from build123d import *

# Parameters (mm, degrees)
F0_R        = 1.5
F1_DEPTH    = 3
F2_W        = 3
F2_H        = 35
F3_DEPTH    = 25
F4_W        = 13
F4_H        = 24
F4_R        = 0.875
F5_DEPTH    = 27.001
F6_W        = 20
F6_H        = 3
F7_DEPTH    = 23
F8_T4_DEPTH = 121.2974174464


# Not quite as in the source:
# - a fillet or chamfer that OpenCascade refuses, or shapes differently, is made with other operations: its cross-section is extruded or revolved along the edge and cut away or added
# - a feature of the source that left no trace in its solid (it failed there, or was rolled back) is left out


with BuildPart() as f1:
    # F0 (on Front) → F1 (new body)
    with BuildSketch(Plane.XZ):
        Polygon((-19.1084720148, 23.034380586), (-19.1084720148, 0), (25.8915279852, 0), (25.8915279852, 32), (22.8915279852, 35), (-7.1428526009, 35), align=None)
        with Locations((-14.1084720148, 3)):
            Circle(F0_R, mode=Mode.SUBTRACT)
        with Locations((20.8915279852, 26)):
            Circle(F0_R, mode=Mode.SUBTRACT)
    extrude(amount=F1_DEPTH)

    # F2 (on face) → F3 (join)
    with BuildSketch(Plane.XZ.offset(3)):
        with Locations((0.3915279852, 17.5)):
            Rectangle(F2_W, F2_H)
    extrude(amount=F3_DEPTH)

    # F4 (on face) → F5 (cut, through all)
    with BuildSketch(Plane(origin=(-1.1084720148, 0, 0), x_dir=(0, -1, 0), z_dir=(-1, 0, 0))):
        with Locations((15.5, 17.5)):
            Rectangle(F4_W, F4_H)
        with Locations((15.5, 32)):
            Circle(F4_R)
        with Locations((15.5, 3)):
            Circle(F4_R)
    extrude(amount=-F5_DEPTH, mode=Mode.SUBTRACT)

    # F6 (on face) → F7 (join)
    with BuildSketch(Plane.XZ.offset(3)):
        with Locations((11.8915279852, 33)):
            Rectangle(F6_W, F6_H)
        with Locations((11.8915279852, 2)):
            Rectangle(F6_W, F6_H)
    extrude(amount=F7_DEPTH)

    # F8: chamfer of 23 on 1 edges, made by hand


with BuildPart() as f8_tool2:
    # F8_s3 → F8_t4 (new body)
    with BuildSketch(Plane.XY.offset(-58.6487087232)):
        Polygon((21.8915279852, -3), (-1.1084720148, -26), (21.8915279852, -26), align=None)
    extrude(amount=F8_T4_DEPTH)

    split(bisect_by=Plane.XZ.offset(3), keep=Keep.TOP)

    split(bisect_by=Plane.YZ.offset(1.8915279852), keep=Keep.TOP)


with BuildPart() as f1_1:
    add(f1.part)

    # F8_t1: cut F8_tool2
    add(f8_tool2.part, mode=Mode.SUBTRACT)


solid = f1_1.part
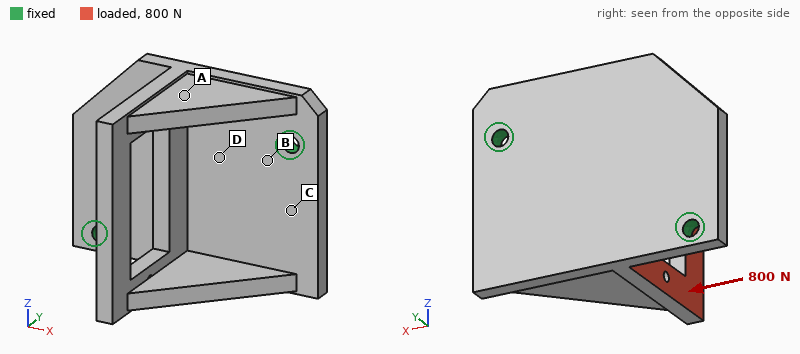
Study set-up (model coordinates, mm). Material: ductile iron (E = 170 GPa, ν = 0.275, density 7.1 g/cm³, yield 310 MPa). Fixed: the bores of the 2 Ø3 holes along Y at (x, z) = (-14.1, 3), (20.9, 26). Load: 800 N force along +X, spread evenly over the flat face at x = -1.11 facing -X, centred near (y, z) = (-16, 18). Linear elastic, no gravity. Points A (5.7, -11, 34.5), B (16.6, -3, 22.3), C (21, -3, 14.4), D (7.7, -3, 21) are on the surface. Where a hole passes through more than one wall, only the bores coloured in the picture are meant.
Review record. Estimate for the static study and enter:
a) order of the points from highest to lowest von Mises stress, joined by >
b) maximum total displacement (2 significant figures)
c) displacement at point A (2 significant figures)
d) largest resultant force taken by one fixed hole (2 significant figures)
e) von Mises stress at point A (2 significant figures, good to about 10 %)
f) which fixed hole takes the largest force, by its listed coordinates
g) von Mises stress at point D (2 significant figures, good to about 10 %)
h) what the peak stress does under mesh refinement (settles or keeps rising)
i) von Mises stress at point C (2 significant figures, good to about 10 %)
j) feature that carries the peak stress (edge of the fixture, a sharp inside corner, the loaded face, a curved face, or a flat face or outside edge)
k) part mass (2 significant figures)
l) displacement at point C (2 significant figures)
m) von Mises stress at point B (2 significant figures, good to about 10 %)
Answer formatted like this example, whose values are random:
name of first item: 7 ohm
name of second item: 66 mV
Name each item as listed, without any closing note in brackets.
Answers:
order of the points from highest to lowest von Mises stress, joined by >: B > C > D > A
maximum total displacement: 0.14 mm
displacement at point A: 0.060 mm
largest resultant force taken by one fixed hole: 530 N
von Mises stress at point A: 17 MPa
which fixed hole takes the largest force, by its listed coordinates: (20.9, 26)
von Mises stress at point D: 32 MPa
what the peak stress does under mesh refinement: keeps rising
von Mises stress at point C: 59 MPa
feature that carries the peak stress: edge of the fixture
part mass: 52 g
displacement at point C: 0.029 mm
von Mises stress at point B: 88 MPa
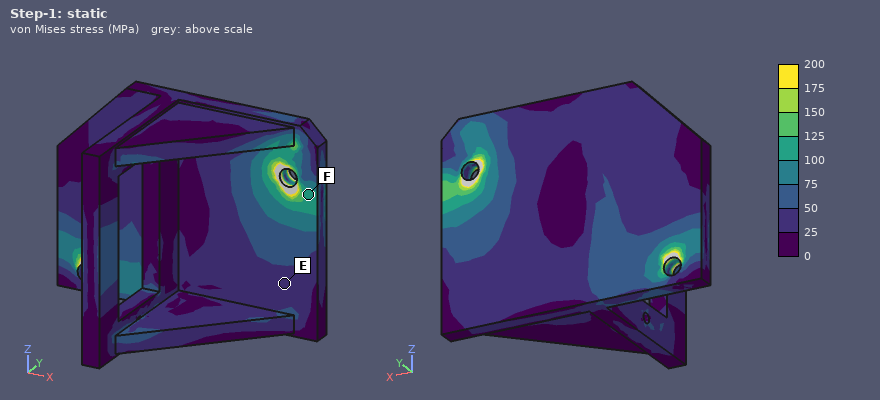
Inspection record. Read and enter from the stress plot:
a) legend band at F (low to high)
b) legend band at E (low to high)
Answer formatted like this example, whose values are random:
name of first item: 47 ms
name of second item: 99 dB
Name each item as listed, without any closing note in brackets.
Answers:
legend band at F: 100 to 125 MPa
legend band at E: 25 to 50 MPa
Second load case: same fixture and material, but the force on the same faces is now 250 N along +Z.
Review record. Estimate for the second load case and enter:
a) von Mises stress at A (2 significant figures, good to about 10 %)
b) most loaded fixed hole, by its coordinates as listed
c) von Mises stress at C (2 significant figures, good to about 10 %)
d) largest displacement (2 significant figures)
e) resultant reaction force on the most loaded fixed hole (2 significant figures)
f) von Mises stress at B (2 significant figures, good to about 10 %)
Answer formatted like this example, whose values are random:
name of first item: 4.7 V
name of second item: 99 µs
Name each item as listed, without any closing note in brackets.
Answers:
von Mises stress at A: 11 MPa
most loaded fixed hole, by its coordinates as listed: (-14.1, 3)
von Mises stress at C: 15 MPa
largest displacement: 54 µm
resultant reaction force on the most loaded fixed hole: 170 N
von Mises stress at B: 29 MPa
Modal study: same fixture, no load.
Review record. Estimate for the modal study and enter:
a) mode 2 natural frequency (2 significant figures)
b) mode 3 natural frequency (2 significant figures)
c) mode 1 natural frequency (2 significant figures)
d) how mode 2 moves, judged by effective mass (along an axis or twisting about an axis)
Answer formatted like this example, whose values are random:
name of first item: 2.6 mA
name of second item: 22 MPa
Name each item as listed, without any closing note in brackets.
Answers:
mode 2 natural frequency: 4200 Hz
mode 3 natural frequency: 5800 Hz
mode 1 natural frequency: 2300 Hz
how mode 2 moves, judged by effective mass: along Y
